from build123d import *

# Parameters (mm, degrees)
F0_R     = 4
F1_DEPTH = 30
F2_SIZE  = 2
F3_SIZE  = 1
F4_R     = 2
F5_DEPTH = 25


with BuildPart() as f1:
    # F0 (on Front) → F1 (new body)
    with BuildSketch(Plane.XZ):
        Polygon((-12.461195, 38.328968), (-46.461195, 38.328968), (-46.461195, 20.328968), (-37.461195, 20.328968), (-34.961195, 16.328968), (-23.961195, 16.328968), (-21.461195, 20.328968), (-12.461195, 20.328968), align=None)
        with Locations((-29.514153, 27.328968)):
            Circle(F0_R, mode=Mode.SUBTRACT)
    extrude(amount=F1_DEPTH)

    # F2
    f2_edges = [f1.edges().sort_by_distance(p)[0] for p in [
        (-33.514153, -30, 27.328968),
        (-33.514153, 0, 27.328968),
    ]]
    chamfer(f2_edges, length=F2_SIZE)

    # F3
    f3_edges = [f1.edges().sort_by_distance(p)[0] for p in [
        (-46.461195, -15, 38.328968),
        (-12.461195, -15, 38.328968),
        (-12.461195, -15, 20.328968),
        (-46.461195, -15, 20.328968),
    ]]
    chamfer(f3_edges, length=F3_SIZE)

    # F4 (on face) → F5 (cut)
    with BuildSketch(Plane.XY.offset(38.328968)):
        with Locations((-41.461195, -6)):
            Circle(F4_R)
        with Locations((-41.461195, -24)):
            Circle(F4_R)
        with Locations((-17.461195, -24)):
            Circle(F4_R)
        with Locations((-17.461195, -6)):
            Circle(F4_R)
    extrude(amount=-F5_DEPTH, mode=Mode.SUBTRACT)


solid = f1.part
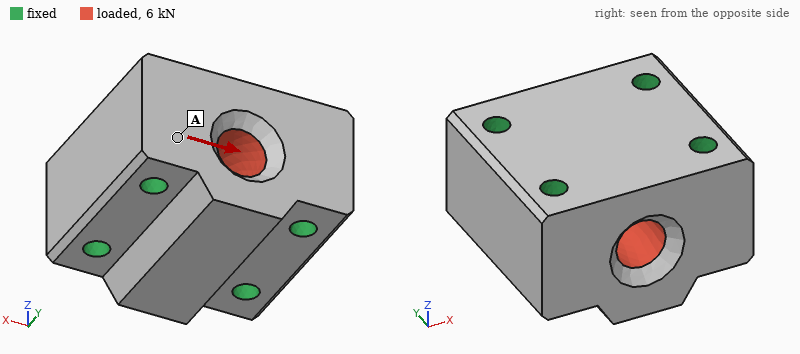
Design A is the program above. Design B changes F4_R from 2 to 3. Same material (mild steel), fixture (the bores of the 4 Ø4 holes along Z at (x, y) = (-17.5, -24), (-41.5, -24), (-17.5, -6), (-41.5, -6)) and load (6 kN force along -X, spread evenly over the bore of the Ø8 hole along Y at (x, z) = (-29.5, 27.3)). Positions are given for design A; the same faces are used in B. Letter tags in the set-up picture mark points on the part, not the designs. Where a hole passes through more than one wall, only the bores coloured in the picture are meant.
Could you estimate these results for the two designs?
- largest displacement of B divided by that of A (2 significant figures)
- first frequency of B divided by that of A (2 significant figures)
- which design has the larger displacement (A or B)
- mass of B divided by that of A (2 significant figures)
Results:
0.85
1.1
A
0.93
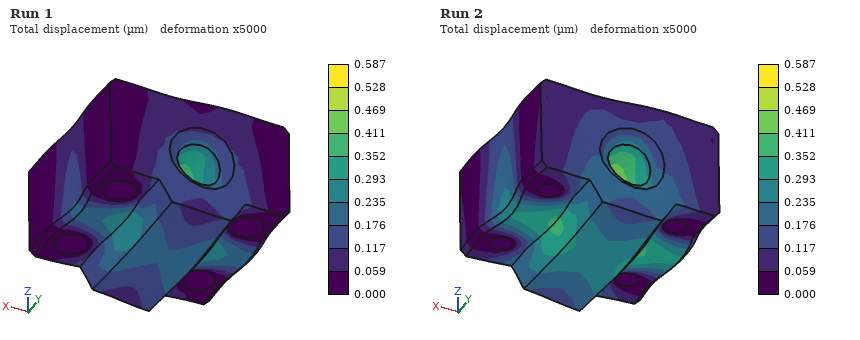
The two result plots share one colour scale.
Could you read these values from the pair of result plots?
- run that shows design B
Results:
Run 1
